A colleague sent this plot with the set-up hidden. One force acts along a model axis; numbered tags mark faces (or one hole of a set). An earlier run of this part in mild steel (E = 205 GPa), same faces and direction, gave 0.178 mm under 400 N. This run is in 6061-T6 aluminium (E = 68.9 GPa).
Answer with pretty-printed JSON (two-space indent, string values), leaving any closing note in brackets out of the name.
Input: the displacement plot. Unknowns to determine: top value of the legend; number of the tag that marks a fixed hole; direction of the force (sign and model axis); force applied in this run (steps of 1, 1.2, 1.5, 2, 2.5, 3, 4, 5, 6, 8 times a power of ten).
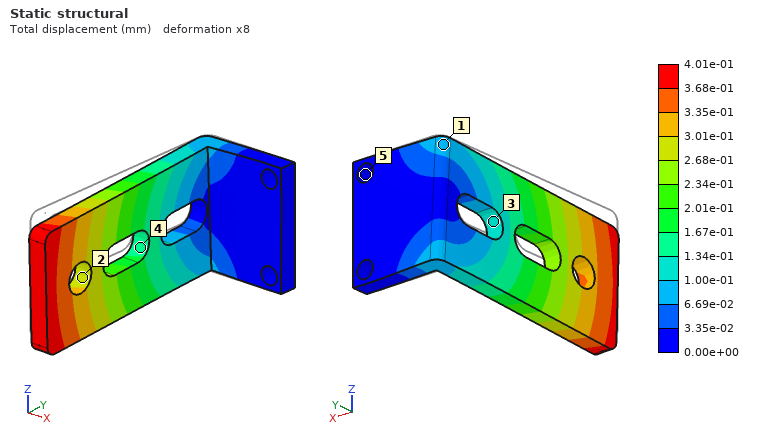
{
  "top value of the legend": "4.01e-01 mm",
  "number of the tag that marks a fixed hole": "5",
  "direction of the force": "-Z",
  "force applied in this run": "300 N"
}
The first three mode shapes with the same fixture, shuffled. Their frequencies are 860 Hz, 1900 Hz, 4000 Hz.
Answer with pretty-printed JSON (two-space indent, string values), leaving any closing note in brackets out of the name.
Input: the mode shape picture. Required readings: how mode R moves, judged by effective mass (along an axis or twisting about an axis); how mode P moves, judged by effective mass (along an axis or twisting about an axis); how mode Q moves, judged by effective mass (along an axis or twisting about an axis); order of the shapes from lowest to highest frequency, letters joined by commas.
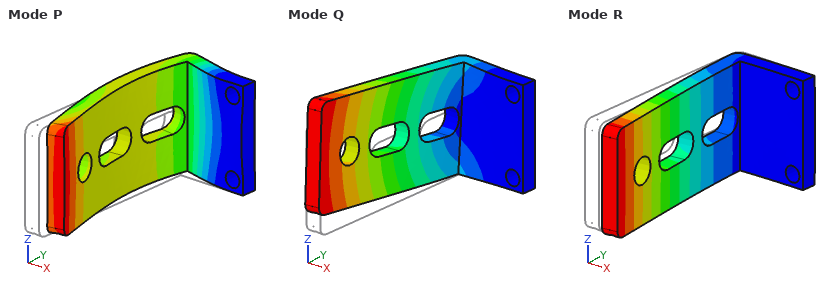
{
  "how mode R moves, judged by effective mass": "along X",
  "how mode P moves, judged by effective mass": "along Y",
  "how mode Q moves, judged by effective mass": "along Z",
  "order of the shapes from lowest to highest frequency, letters joined by commas": "R, Q, P"
}
